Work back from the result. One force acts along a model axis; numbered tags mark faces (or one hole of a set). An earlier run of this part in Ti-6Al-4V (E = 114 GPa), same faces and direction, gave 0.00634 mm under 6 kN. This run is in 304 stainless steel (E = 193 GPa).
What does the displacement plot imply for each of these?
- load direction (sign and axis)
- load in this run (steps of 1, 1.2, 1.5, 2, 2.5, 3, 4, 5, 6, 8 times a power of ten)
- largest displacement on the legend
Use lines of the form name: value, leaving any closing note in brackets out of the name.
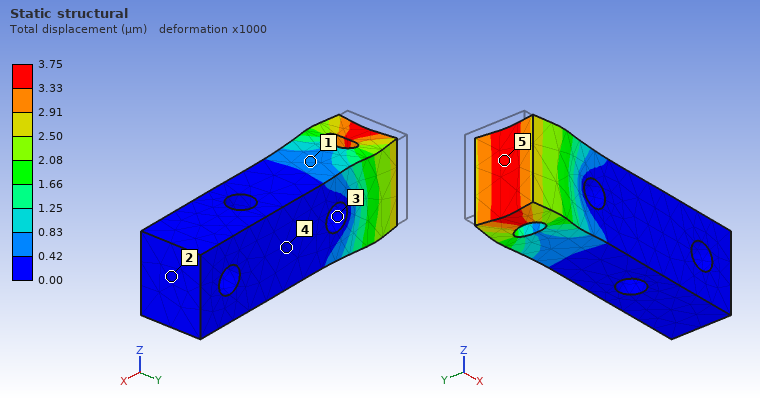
load direction: +X
load in this run: 6 kN
largest displacement on the legend: 3.75 µm
